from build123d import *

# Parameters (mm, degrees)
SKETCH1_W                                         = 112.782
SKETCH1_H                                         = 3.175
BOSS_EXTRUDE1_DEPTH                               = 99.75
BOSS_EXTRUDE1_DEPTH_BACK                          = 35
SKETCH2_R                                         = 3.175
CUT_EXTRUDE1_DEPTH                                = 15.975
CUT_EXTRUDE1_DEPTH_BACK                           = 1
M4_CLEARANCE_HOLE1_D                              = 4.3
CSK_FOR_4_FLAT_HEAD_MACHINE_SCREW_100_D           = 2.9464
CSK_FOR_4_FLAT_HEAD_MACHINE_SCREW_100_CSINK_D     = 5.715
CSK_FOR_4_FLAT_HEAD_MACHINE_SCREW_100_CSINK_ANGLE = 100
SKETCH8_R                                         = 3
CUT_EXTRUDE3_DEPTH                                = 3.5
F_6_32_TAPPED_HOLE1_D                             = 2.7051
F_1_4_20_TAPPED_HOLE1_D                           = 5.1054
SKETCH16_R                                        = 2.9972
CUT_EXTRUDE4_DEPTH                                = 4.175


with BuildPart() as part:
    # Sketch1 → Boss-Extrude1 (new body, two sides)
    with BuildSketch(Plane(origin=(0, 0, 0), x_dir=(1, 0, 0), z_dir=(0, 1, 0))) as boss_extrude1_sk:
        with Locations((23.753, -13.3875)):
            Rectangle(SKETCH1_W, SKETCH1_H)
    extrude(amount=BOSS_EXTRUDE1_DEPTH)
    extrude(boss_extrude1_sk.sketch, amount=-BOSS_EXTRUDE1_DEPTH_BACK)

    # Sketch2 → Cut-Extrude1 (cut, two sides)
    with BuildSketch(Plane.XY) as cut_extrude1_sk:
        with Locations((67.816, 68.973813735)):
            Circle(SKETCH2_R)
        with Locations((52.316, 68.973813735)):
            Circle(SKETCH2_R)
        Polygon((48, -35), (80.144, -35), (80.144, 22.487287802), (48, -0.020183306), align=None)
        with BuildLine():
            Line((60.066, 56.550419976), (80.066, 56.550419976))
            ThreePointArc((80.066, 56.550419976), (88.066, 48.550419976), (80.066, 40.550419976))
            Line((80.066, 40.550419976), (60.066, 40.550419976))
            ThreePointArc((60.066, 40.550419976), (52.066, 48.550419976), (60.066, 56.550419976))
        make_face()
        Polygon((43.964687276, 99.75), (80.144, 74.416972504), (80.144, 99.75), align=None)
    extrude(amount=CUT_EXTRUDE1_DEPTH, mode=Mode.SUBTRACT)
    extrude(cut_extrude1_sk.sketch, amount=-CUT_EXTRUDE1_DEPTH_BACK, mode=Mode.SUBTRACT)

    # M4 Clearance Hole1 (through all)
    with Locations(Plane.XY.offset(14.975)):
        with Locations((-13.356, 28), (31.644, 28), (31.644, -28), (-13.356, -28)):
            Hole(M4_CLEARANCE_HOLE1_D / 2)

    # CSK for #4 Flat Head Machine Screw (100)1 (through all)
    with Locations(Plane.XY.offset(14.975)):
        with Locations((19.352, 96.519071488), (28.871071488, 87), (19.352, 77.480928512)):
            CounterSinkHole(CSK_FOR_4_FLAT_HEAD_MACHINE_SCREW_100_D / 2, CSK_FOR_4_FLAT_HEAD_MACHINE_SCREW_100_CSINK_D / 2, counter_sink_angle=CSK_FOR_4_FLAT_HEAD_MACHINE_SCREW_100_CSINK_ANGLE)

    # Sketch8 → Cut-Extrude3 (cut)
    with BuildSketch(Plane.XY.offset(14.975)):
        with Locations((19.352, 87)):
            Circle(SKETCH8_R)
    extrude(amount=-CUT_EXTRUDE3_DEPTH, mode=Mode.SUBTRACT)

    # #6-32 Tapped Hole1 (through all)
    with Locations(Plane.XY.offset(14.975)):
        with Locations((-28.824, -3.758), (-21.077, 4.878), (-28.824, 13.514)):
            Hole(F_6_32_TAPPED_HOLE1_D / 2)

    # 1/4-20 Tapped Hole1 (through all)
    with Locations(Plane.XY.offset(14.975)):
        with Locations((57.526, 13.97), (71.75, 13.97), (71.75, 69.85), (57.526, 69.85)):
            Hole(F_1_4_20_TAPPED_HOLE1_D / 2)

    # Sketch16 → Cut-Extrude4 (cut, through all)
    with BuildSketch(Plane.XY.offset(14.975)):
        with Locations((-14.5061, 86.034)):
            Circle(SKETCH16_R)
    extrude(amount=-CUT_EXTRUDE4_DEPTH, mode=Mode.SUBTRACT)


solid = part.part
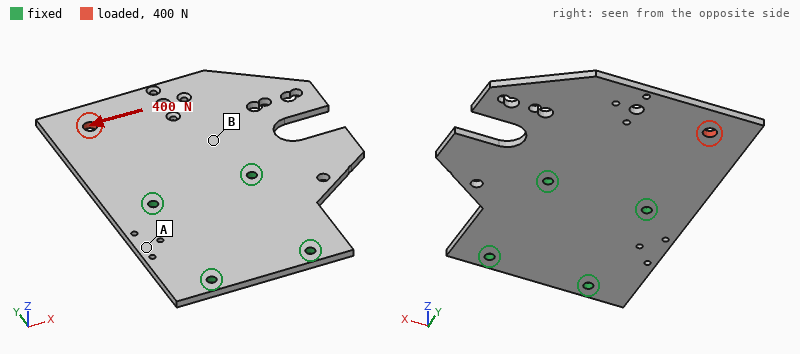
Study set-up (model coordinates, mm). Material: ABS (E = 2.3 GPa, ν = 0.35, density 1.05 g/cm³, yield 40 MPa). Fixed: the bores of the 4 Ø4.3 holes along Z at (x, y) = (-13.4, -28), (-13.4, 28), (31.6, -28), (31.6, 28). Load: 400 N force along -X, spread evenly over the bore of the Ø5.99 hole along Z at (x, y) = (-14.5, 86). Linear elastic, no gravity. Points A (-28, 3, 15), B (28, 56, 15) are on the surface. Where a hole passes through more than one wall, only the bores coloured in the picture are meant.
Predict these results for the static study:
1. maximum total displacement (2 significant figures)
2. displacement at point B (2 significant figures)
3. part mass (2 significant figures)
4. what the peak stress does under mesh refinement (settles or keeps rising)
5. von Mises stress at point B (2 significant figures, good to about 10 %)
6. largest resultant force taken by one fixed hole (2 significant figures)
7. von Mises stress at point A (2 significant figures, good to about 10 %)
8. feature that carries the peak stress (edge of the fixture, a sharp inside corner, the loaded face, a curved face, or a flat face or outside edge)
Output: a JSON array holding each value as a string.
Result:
["0.35 mm", "0.11 mm", "42 g", "keeps rising", "3.5 MPa", "420 N", "1.6 MPa", "edge of the fixture"]
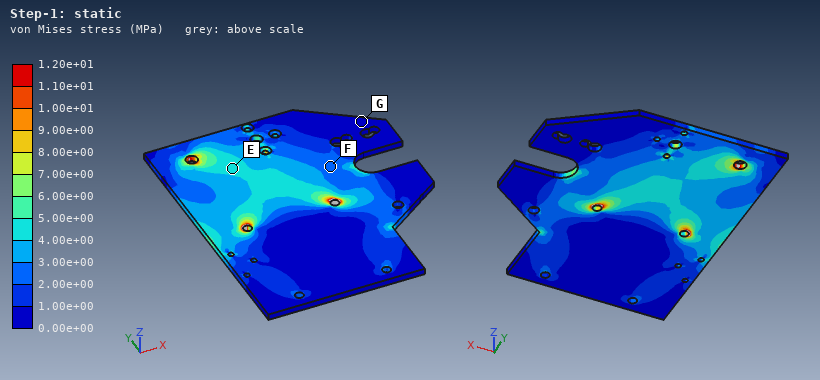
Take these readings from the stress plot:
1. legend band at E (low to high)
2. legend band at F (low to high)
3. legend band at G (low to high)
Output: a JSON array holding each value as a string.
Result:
["4.00e+00 to 5.00e+00 MPa", "2.00e+00 to 3.00e+00 MPa", "0.00e+00 to 1.00e+00 MPa"]
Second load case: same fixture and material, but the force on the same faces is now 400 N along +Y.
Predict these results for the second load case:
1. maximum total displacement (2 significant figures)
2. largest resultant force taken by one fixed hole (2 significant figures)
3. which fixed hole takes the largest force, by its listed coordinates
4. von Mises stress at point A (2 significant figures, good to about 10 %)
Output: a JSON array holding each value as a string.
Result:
["0.15 mm", "300 N", "(-13.4, 28)", "0.94 MPa"]
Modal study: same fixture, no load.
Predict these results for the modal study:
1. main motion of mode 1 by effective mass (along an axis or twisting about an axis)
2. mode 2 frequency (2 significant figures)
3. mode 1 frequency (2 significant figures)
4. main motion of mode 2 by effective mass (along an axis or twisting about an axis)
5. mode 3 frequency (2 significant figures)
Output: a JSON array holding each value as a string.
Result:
["along Z", "240 Hz", "140 Hz", "twisting about Y", "440 Hz"]
